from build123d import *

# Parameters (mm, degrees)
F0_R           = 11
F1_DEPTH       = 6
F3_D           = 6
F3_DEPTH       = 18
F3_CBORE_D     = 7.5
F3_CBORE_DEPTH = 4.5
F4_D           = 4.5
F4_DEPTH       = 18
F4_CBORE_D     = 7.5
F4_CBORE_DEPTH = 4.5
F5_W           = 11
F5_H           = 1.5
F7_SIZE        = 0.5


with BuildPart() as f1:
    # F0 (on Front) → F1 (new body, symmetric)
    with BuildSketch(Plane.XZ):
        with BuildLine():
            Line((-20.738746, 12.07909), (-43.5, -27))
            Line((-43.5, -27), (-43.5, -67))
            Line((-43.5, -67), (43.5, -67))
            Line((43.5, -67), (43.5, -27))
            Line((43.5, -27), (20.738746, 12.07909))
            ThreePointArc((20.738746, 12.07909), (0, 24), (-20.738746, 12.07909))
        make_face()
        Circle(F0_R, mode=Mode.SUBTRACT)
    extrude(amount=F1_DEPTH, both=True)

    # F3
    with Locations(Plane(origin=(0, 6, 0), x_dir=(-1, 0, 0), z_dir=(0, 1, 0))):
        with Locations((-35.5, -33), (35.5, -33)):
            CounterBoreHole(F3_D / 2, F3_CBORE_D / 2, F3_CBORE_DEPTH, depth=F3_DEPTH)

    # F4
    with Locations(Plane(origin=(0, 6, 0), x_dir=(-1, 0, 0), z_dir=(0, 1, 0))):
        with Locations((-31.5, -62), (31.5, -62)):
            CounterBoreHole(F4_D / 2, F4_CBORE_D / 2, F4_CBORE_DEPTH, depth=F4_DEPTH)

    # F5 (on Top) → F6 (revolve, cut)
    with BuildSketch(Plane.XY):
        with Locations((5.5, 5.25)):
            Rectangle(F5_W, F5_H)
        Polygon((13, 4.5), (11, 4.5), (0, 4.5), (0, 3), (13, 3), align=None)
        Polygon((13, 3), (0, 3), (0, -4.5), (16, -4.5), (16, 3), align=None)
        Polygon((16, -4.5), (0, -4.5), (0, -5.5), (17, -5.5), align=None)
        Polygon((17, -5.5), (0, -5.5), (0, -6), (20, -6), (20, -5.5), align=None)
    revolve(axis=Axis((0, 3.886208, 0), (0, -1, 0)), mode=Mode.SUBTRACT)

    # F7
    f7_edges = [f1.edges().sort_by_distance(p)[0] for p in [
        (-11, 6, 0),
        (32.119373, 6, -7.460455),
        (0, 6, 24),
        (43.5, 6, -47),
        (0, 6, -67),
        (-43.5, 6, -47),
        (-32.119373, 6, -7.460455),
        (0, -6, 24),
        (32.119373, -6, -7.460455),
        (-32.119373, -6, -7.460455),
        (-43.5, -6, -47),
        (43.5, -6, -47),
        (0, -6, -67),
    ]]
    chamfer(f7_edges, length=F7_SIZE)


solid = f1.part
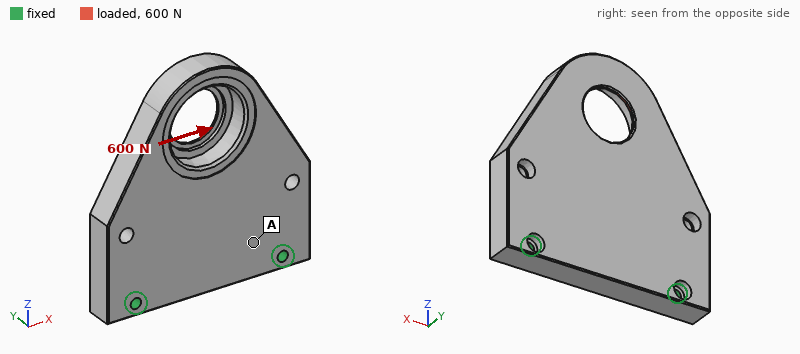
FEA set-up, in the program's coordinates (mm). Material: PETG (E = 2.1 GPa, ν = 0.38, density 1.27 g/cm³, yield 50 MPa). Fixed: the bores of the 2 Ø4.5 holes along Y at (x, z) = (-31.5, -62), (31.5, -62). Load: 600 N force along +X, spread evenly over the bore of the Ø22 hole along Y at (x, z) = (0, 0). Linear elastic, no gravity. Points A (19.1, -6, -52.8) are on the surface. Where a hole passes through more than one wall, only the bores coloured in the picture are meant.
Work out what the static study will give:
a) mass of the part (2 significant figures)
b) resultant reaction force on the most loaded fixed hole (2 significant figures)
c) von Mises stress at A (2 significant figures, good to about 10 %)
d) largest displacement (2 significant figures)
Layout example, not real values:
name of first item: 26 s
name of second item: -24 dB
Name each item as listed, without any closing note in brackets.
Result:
mass of the part: 83 g
resultant reaction force on the most loaded fixed hole: 650 N
von Mises stress at A: 2.0 MPa
largest displacement: 0.28 mm
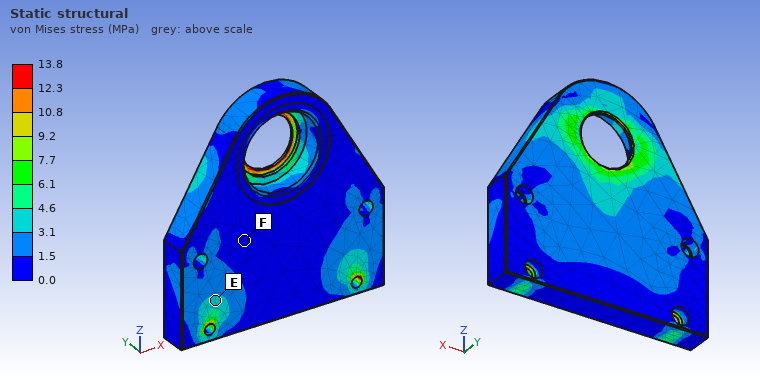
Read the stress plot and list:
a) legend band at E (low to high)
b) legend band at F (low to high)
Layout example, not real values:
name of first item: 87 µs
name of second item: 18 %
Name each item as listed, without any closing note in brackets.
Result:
legend band at E: 3.1 to 4.6 MPa
legend band at F: 0.0 to 1.5 MPa
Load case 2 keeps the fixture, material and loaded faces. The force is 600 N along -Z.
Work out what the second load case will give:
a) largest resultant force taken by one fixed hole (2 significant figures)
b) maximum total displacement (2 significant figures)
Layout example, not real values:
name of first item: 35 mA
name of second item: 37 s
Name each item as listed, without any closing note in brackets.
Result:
largest resultant force taken by one fixed hole: 310 N
maximum total displacement: 1.1 mm
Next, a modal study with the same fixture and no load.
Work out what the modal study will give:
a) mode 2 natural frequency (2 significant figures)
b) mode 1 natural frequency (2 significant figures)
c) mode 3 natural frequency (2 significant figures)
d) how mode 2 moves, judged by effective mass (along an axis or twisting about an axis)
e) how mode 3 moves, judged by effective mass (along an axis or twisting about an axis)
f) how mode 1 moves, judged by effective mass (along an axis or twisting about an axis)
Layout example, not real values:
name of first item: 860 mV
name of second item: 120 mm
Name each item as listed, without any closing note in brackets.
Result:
mode 2 natural frequency: 1100 Hz
mode 1 natural frequency: 320 Hz
mode 3 natural frequency: 1600 Hz
how mode 2 moves, judged by effective mass: twisting about Z
how mode 3 moves, judged by effective mass: along Y
how mode 1 moves, judged by effective mass: along Y
